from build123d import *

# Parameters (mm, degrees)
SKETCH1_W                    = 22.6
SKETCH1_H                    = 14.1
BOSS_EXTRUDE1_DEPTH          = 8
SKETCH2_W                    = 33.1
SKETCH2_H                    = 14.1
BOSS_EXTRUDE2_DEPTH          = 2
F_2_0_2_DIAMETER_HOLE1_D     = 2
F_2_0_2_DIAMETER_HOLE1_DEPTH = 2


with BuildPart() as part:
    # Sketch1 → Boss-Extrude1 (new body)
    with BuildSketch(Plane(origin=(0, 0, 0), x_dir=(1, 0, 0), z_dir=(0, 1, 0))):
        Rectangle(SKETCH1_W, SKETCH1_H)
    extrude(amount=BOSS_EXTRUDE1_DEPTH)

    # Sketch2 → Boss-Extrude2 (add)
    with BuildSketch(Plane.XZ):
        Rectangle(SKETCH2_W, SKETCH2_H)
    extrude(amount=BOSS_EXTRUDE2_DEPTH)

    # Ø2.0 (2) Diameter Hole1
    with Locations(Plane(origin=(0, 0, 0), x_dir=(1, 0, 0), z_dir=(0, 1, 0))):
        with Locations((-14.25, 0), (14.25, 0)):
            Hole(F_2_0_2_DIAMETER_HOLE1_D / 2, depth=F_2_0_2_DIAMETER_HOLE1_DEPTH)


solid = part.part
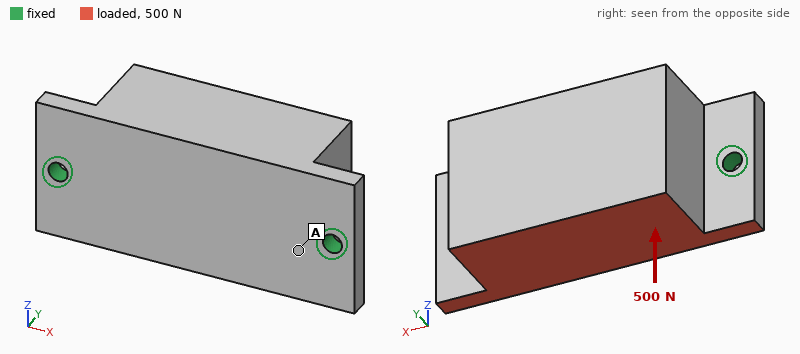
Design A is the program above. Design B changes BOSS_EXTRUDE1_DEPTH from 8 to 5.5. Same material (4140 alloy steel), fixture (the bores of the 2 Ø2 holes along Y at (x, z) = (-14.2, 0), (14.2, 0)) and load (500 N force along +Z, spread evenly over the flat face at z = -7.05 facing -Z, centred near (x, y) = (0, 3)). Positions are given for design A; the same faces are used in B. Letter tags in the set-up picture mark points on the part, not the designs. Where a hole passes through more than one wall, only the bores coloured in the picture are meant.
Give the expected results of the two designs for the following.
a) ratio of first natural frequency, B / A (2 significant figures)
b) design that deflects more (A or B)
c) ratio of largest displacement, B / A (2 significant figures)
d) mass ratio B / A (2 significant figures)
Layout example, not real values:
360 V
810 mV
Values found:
1.4
A
0.60
0.77
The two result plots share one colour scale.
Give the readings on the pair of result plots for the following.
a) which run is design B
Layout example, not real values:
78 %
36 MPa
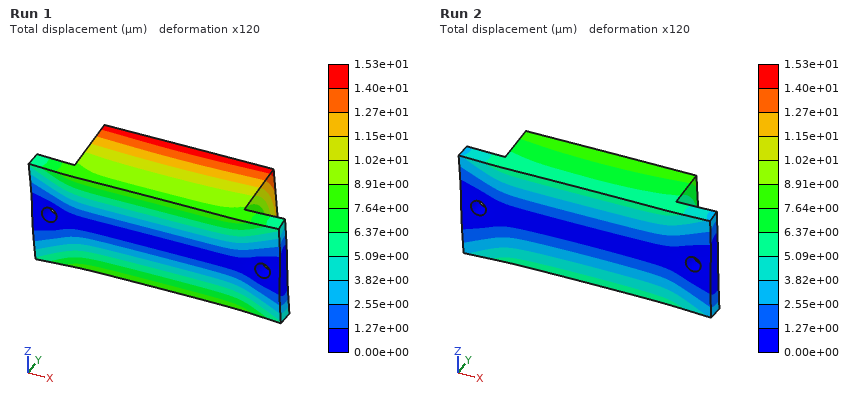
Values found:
Run 2
